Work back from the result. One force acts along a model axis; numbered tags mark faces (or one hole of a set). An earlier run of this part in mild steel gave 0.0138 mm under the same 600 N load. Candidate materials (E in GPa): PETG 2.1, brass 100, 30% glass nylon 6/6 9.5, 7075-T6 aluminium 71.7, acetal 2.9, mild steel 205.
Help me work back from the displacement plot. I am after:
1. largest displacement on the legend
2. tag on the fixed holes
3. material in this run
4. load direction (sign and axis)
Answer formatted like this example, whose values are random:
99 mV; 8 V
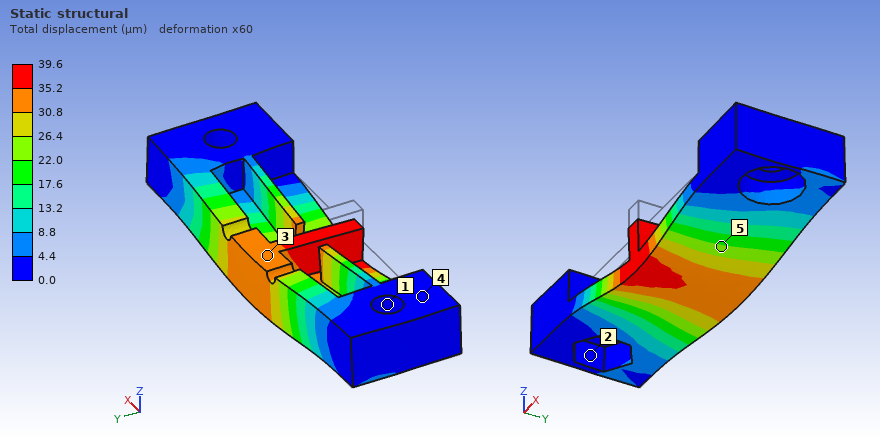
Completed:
39.6 µm; 1; 7075-T6 aluminium; -Z
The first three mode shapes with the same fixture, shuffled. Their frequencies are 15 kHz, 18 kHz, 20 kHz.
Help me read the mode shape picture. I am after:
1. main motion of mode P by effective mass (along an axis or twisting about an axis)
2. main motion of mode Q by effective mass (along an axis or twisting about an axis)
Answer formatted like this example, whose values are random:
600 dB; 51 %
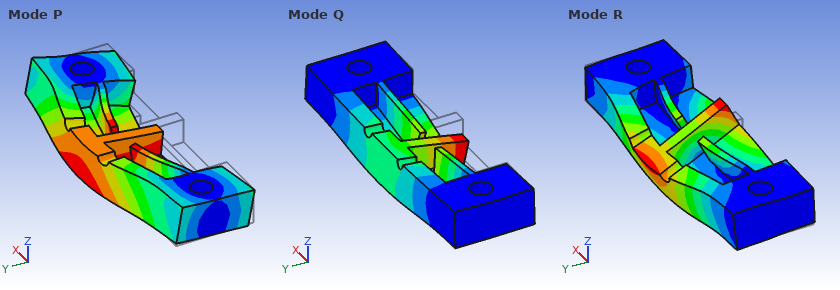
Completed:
along Y; along Z
